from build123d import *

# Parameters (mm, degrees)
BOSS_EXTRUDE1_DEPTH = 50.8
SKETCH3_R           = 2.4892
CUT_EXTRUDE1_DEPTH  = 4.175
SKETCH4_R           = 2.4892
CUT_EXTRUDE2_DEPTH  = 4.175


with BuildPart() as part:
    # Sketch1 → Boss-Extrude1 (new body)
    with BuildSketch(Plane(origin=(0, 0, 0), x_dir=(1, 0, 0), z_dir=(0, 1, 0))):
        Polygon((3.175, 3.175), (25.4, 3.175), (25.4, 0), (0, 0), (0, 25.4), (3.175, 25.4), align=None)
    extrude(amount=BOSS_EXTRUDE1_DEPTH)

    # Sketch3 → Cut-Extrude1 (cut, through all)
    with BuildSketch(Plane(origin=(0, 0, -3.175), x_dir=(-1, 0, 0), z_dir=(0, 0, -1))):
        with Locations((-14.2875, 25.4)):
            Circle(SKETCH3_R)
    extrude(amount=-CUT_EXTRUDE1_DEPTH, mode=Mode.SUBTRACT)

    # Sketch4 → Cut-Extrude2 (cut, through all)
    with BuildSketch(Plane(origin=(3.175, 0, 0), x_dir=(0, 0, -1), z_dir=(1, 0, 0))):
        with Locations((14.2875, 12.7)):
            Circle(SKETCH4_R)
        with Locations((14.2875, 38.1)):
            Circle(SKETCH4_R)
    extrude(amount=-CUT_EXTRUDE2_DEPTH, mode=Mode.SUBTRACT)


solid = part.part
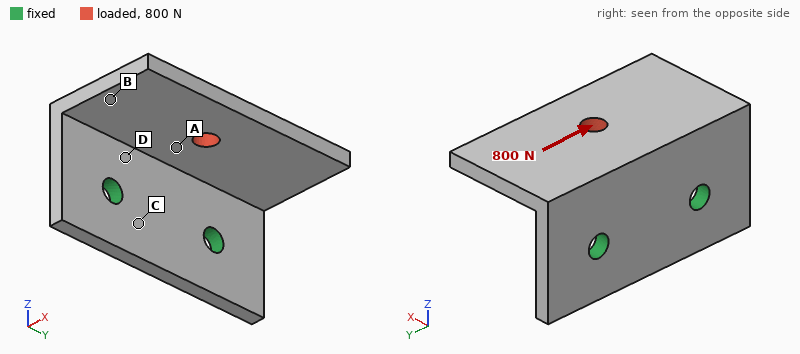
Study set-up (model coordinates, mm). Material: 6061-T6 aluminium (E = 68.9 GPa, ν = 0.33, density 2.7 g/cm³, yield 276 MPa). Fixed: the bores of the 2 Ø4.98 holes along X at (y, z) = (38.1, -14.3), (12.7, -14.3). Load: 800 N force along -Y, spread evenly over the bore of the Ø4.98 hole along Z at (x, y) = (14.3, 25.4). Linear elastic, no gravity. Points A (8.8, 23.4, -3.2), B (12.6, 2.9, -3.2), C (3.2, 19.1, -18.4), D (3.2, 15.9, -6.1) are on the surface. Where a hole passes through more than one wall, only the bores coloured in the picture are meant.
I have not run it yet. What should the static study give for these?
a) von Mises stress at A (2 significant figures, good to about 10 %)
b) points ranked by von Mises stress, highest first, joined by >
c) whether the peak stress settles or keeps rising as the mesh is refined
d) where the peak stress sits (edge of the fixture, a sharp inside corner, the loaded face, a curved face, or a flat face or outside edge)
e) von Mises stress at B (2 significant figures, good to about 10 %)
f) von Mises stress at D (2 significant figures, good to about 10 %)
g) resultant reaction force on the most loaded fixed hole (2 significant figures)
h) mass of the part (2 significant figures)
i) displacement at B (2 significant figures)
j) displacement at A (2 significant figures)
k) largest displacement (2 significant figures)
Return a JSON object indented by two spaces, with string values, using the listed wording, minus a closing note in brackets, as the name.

{
  "von Mises stress at A": "31 MPa",
  "points ranked by von Mises stress, highest first, joined by >": "D > A > B > C",
  "whether the peak stress settles or keeps rising as the mesh is refined": "keeps rising",
  "where the peak stress sits": "edge of the fixture",
  "von Mises stress at B": "16 MPa",
  "von Mises stress at D": "42 MPa",
  "resultant reaction force on the most loaded fixed hole": "620 N",
  "mass of the part": "20 g",
  "displacement at B": "57 µm",
  "displacement at A": "21 µm",
  "largest displacement": "89 µm"
}
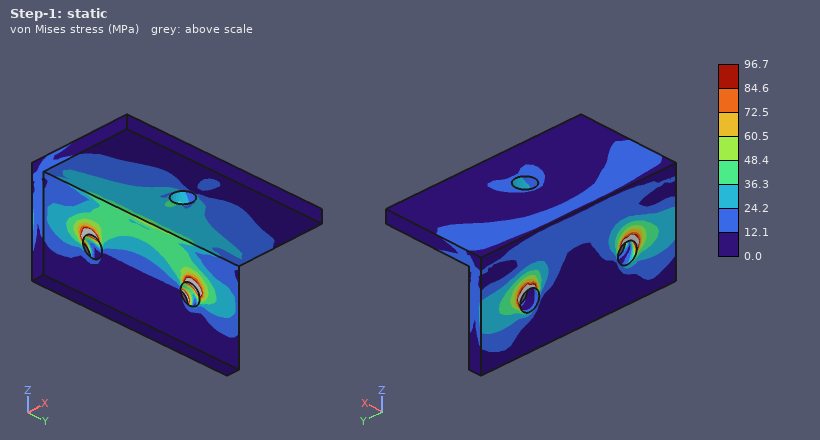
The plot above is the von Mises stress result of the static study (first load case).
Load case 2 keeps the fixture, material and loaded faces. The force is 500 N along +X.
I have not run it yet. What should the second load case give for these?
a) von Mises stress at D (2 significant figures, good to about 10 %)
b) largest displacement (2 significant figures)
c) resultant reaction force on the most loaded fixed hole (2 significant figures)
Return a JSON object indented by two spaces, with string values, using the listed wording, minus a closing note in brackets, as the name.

{
  "von Mises stress at D": "27 MPa",
  "largest displacement": "0.10 mm",
  "resultant reaction force on the most loaded fixed hole": "250 N"
}
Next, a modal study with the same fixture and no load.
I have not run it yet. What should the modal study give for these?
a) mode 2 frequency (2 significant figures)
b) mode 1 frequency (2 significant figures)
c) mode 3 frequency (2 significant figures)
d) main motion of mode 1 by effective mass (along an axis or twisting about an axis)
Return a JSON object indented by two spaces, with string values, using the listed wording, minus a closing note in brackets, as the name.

{
  "mode 2 frequency": "4300 Hz",
  "mode 1 frequency": "2600 Hz",
  "mode 3 frequency": "7000 Hz",
  "main motion of mode 1 by effective mass": "along Z"
}
